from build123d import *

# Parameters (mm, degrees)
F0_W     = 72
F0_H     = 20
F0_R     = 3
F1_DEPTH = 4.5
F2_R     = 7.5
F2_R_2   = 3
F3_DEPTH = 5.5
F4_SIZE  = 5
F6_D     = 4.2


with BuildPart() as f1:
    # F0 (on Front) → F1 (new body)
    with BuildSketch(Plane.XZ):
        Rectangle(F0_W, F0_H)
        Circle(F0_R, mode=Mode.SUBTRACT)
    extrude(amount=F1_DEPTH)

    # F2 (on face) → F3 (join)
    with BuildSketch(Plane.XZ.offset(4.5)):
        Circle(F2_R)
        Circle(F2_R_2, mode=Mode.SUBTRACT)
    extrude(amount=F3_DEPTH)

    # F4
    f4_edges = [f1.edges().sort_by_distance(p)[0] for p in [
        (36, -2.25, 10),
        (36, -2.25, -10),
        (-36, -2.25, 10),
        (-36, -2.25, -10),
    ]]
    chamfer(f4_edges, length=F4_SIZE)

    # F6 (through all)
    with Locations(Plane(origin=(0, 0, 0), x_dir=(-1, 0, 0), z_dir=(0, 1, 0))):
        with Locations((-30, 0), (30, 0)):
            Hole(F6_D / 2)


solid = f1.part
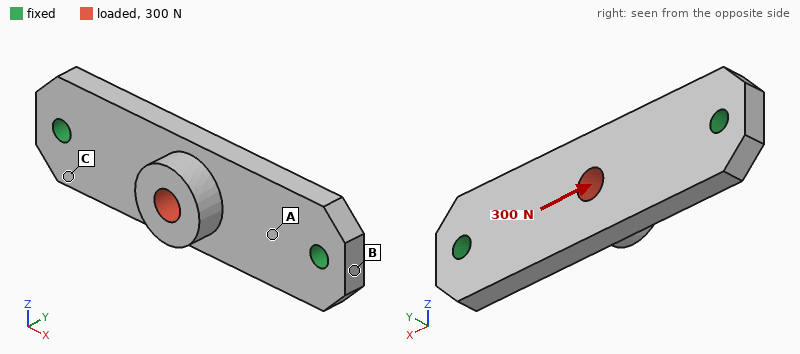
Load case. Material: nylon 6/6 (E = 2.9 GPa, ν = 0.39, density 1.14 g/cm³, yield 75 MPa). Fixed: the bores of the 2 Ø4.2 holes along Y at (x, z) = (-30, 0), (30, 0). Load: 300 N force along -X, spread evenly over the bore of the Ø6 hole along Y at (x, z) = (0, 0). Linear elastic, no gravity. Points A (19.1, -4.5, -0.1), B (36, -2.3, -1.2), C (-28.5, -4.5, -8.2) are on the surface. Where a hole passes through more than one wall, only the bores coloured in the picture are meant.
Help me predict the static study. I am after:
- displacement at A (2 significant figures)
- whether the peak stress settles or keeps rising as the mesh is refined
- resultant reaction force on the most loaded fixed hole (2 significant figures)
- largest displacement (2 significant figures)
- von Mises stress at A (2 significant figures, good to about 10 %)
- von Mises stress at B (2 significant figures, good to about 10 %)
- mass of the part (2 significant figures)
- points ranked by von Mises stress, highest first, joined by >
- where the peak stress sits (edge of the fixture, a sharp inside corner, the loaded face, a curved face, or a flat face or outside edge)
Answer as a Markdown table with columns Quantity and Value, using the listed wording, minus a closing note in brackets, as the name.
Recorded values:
| Quantity | Value |
|---|---|
| displacement at A | 17 µm |
| whether the peak stress settles or keeps rising as the mesh is refined | keeps rising |
| resultant reaction force on the most loaded fixed hole | 150 N |
| largest displacement | 57 µm |
| von Mises stress at A | 2.9 MPa |
| von Mises stress at B | 1.9 MPa |
| mass of the part | 7.8 g |
| points ranked by von Mises stress, highest first, joined by > | A > B > C |
| where the peak stress sits | edge of the fixture |
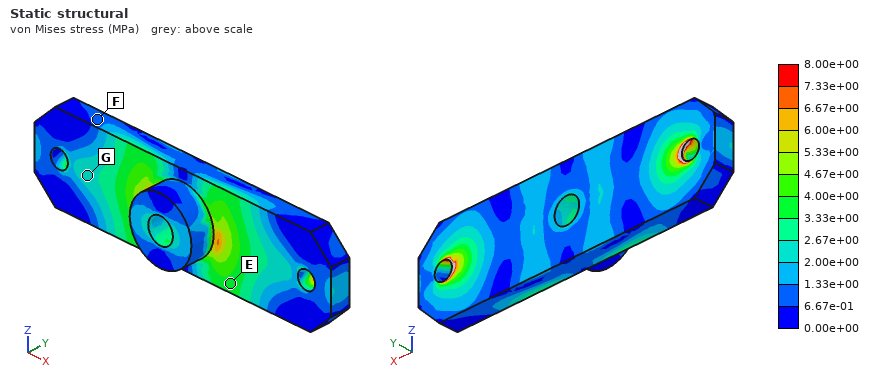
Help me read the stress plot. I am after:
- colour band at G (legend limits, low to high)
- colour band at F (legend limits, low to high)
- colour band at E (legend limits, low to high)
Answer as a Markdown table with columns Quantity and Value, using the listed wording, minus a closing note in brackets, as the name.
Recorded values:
| Quantity | Value |
|---|---|
| colour band at G | 2.00e+00 to 2.67e+00 MPa |
| colour band at F | 6.67e-01 to 1.33e+00 MPa |
| colour band at E | 3.33e+00 to 4.00e+00 MPa |
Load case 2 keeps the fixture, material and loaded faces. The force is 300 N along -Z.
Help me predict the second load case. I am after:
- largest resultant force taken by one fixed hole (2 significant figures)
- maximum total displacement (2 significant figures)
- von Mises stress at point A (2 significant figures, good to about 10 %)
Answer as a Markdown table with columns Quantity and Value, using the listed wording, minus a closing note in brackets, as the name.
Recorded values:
| Quantity | Value |
|---|---|
| largest resultant force taken by one fixed hole | 150 N |
| maximum total displacement | 0.30 mm |
| von Mises stress at point A | 9.8 MPa |
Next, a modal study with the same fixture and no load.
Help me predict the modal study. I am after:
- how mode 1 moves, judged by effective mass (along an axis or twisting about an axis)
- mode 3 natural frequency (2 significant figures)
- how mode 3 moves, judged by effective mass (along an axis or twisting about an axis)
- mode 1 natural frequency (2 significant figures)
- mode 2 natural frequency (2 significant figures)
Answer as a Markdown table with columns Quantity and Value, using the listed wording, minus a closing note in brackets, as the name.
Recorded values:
| Quantity | Value |
|---|---|
| how mode 1 moves, judged by effective mass | along Y |
| mode 3 natural frequency | 4000 Hz |
| how mode 3 moves, judged by effective mass | along Z |
| mode 1 natural frequency | 1900 Hz |
| mode 2 natural frequency | 2800 Hz |
